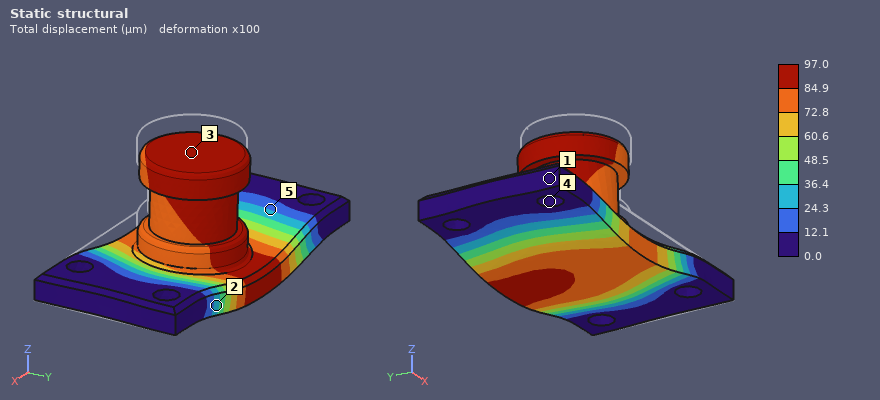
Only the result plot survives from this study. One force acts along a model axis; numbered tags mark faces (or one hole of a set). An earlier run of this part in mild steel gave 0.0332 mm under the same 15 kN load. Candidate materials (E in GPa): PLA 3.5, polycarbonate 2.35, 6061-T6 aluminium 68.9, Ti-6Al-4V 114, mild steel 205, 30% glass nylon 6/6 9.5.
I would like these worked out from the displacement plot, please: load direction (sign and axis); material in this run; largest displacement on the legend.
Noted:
-Z
6061-T6 aluminium
97.0 µm
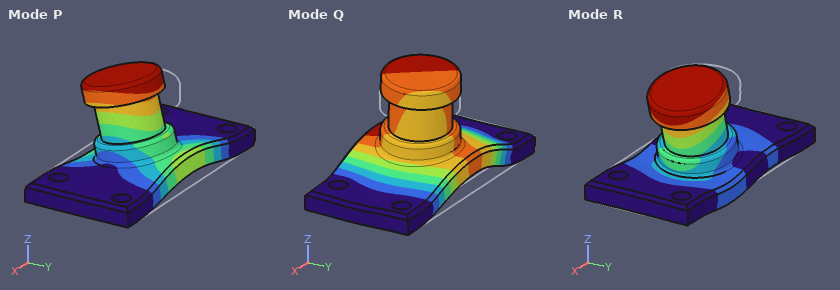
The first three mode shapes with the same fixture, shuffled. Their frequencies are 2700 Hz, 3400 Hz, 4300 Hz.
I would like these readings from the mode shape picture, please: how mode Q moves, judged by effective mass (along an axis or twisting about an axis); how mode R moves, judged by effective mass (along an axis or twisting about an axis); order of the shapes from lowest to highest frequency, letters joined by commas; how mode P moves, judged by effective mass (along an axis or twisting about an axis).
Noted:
along Z
along X
P, Q, R
along Y
